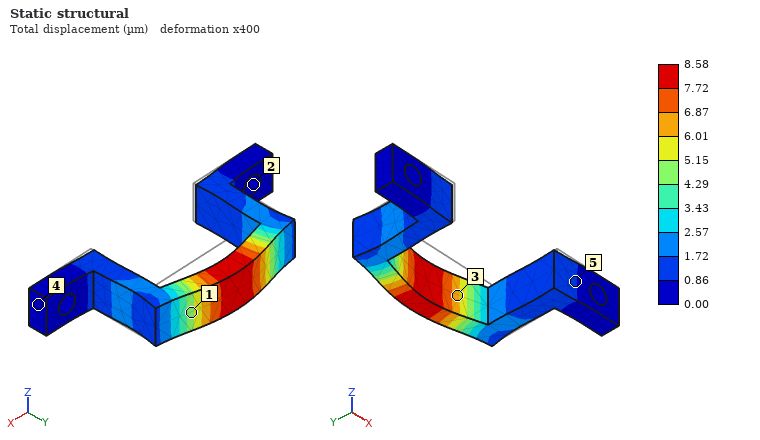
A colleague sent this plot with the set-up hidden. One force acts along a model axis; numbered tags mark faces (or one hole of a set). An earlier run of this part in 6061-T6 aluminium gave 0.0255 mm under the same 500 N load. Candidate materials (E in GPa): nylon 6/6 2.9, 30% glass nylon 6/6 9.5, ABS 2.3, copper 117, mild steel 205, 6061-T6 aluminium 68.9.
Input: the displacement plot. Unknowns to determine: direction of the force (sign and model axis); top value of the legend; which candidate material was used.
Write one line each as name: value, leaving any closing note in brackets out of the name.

direction of the force: +Y
top value of the legend: 8.58 µm
which candidate material was used: mild steel
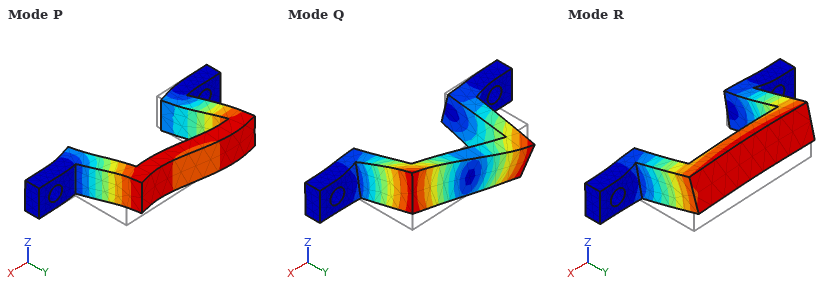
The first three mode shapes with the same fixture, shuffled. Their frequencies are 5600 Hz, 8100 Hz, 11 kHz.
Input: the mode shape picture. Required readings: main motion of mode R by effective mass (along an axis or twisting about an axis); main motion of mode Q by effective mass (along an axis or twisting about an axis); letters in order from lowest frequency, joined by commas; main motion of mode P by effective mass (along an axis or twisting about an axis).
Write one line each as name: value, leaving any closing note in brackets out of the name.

main motion of mode R by effective mass: along Z
main motion of mode Q by effective mass: twisting about Y
letters in order from lowest frequency, joined by commas: R, P, Q
main motion of mode P by effective mass: along X
